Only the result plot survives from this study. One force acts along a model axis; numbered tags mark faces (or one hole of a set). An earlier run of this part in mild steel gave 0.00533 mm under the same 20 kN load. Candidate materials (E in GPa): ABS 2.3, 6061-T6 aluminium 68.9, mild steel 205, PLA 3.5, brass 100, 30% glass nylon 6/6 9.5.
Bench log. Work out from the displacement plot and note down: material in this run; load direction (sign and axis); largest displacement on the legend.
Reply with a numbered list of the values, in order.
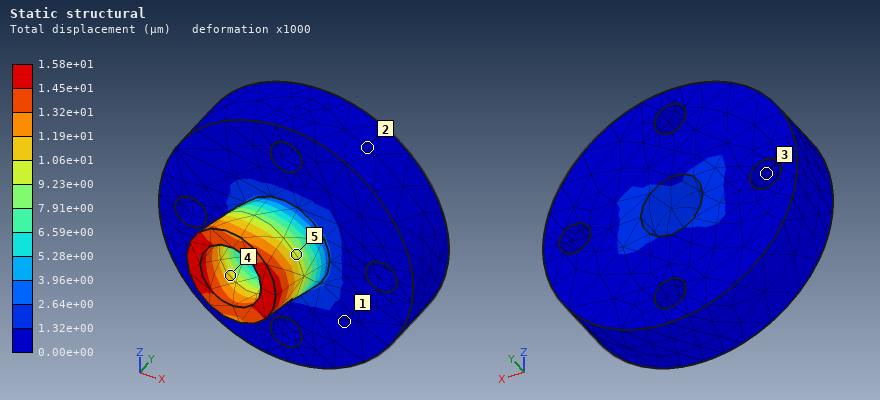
1. 6061-T6 aluminium
2. -X
3. 1.58e+01 µm
